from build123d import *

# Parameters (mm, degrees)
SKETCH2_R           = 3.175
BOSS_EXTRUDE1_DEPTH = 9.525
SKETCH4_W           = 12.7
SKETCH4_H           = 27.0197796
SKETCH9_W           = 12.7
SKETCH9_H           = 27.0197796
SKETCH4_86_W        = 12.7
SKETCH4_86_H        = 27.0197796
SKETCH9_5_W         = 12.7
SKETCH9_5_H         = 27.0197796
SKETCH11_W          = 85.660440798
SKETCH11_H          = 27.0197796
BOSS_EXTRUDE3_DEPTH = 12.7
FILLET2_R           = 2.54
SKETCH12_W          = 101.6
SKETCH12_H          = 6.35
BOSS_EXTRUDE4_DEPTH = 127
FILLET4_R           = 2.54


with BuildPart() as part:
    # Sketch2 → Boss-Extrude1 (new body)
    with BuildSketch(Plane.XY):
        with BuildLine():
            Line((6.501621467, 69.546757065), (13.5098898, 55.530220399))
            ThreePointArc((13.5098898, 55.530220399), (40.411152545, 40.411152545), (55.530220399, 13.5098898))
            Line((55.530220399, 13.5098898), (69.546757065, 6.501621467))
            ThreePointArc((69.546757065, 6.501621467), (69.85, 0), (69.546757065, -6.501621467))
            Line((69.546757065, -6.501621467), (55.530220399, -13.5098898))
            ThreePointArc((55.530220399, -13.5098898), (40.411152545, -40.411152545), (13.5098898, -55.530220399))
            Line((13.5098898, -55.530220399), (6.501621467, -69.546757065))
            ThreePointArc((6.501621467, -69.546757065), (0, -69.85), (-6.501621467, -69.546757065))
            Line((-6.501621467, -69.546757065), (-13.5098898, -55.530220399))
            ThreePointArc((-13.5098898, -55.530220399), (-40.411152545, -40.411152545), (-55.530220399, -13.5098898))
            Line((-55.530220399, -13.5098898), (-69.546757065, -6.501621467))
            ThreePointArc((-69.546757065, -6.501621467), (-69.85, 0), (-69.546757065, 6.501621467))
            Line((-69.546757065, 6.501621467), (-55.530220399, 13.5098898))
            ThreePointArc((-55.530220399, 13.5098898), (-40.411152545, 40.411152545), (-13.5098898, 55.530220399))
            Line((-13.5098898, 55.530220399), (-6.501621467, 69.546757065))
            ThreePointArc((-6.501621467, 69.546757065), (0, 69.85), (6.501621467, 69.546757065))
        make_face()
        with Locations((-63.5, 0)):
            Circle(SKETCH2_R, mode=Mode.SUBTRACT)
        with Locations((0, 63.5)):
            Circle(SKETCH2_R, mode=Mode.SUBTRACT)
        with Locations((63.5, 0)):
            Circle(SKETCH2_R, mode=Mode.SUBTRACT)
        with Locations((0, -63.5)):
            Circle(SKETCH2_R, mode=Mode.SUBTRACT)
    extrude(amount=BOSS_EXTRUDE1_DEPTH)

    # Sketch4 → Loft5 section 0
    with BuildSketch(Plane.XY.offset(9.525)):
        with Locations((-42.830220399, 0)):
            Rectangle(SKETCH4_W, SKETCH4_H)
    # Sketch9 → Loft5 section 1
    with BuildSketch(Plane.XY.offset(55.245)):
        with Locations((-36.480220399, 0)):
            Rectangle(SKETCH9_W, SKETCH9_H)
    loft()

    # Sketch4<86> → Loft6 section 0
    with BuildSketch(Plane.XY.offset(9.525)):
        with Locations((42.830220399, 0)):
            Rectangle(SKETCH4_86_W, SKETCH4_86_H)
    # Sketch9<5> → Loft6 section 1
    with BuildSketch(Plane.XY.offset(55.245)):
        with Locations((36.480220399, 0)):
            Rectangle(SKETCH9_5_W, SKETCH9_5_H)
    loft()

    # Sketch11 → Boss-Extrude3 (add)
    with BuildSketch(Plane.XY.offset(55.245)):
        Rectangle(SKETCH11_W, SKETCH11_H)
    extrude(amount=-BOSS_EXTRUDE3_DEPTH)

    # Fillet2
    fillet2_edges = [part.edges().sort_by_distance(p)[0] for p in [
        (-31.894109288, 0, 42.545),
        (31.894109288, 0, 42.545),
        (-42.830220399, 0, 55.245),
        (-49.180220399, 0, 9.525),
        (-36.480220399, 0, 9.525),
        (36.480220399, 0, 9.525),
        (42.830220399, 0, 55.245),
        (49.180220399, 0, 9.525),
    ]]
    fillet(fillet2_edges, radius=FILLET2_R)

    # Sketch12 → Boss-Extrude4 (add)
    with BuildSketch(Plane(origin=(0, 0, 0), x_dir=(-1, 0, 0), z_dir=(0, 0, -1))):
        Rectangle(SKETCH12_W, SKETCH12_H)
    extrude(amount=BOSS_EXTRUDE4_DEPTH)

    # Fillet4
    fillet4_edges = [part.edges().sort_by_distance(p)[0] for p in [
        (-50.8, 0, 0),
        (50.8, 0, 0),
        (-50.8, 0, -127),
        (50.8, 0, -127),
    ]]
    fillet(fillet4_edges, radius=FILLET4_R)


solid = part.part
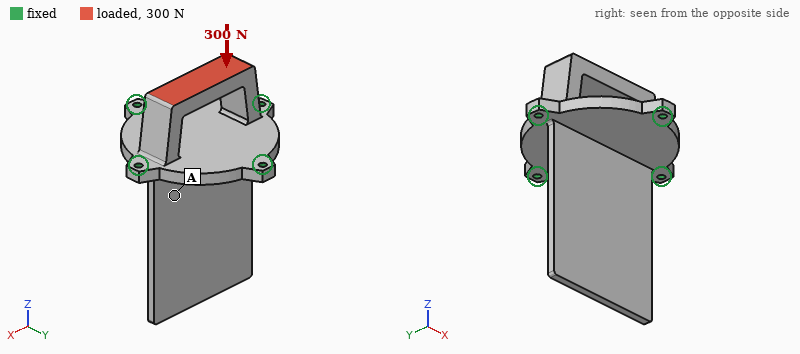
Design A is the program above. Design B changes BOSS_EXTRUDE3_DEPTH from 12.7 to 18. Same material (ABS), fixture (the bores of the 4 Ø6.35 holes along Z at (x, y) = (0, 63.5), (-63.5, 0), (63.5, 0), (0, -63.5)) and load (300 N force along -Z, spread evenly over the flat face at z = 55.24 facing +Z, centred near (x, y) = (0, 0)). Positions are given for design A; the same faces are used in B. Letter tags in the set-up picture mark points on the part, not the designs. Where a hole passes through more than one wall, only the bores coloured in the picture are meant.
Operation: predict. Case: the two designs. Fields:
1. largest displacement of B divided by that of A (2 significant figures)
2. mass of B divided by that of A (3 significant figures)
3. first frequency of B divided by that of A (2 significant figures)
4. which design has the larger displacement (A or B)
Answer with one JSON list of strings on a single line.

["0.71", "1.04", "1.0", "A"]
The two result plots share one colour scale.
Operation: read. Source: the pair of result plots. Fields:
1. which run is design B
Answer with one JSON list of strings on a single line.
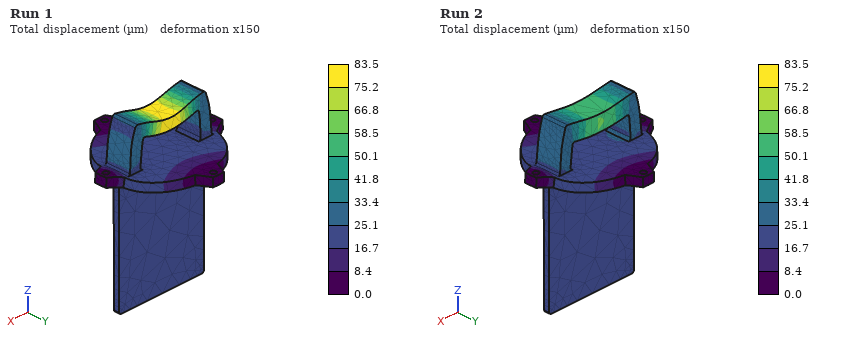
["Run 2"]
